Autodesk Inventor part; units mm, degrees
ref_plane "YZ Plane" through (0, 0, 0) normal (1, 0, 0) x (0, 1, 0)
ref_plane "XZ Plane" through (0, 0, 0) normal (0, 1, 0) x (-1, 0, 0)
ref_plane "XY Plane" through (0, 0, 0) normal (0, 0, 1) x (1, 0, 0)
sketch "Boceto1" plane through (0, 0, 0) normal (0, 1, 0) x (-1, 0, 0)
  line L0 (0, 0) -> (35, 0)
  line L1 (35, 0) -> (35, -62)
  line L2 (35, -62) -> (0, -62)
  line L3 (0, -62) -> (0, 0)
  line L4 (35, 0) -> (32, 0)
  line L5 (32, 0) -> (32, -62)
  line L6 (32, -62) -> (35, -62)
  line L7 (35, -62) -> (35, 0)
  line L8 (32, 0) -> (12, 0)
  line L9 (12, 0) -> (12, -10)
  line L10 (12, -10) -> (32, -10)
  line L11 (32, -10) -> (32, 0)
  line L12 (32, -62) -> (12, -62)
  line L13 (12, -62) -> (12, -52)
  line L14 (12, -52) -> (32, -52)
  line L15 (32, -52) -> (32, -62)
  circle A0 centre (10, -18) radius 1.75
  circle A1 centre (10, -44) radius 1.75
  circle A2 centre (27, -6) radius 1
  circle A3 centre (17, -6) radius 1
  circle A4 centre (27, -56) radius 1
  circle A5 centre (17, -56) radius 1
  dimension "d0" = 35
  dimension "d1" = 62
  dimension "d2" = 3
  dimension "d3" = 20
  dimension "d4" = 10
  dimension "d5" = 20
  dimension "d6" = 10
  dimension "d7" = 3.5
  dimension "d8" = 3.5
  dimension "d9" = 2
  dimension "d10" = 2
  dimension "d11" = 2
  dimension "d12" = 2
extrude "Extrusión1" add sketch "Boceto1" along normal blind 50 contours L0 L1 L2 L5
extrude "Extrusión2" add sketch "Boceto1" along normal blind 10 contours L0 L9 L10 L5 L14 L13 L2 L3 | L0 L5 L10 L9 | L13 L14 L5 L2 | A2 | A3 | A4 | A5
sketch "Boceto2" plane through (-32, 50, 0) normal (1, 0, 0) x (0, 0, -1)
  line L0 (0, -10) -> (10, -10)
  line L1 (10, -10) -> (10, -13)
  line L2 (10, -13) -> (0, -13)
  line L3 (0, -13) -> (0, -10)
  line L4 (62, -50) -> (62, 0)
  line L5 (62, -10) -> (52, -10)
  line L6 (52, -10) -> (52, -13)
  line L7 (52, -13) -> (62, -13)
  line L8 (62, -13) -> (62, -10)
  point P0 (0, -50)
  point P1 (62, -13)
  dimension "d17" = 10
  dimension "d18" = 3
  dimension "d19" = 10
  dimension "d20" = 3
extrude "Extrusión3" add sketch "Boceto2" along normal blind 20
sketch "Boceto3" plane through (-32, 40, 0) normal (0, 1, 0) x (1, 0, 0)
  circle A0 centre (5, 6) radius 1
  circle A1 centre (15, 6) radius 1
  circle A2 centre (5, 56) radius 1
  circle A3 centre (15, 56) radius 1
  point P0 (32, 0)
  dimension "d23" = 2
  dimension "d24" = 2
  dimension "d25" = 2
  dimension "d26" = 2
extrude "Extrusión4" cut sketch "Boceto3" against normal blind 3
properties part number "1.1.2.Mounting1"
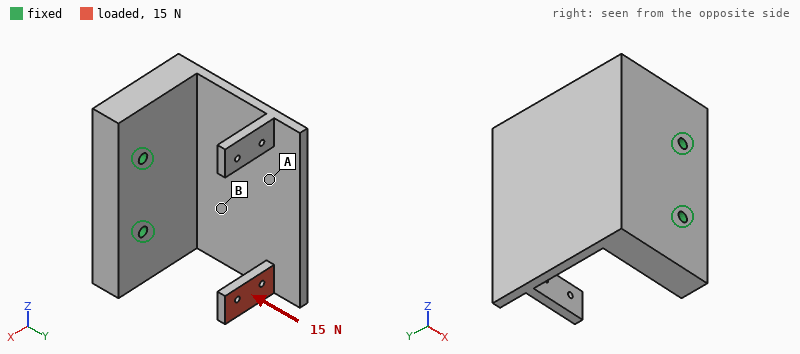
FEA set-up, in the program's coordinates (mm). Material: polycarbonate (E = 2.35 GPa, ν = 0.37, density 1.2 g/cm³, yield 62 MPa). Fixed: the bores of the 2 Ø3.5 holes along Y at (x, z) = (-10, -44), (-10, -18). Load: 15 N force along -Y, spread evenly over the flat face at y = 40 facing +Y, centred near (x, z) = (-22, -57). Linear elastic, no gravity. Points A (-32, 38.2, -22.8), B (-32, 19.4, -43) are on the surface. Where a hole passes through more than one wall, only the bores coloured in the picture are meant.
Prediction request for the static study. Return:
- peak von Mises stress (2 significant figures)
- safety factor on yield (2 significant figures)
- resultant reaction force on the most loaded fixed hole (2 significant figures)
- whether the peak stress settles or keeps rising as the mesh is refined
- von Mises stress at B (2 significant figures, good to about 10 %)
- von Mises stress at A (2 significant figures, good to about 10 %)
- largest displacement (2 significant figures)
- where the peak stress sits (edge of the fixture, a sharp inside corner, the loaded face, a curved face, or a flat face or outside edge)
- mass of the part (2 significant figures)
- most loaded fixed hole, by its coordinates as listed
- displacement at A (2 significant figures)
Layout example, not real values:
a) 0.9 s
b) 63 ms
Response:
a) 14 MPa
b) 4.6
c) 18 N
d) settles
e) 2.3 MPa
f) 1.1 MPa
g) 0.99 mm
h) the loaded face
i) 36 g
j) (-10, -44)
k) 0.17 mm
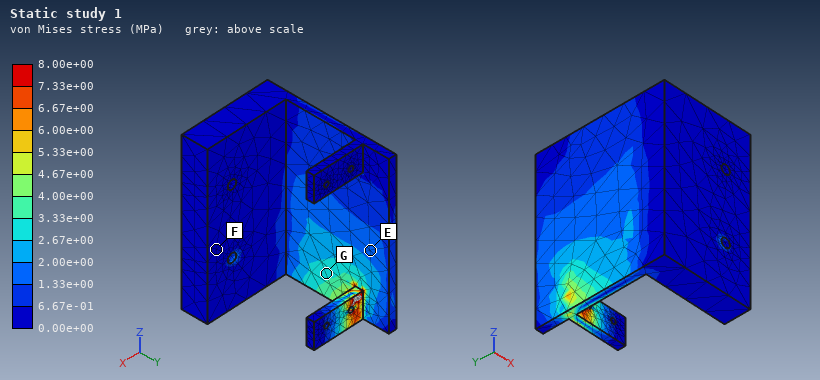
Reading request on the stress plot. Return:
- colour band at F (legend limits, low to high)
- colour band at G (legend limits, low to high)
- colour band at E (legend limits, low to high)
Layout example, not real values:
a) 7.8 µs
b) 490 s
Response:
a) 0.00e+00 to 6.67e-01 MPa
b) 2.67e+00 to 3.33e+00 MPa
c) 1.33e+00 to 2.00e+00 MPa
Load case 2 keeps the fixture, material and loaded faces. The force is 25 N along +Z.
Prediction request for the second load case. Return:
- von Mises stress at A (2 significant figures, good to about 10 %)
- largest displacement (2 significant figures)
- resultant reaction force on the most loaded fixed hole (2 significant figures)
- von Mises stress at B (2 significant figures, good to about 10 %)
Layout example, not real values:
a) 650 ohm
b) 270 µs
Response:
a) 1.1 MPa
b) 0.87 mm
c) 31 N
d) 2.5 MPa
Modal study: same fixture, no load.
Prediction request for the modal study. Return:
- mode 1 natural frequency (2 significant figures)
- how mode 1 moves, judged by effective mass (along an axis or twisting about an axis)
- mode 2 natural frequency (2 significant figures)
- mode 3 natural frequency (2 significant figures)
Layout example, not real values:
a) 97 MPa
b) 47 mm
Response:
a) 350 Hz
b) along X
c) 540 Hz
d) 1000 Hz
